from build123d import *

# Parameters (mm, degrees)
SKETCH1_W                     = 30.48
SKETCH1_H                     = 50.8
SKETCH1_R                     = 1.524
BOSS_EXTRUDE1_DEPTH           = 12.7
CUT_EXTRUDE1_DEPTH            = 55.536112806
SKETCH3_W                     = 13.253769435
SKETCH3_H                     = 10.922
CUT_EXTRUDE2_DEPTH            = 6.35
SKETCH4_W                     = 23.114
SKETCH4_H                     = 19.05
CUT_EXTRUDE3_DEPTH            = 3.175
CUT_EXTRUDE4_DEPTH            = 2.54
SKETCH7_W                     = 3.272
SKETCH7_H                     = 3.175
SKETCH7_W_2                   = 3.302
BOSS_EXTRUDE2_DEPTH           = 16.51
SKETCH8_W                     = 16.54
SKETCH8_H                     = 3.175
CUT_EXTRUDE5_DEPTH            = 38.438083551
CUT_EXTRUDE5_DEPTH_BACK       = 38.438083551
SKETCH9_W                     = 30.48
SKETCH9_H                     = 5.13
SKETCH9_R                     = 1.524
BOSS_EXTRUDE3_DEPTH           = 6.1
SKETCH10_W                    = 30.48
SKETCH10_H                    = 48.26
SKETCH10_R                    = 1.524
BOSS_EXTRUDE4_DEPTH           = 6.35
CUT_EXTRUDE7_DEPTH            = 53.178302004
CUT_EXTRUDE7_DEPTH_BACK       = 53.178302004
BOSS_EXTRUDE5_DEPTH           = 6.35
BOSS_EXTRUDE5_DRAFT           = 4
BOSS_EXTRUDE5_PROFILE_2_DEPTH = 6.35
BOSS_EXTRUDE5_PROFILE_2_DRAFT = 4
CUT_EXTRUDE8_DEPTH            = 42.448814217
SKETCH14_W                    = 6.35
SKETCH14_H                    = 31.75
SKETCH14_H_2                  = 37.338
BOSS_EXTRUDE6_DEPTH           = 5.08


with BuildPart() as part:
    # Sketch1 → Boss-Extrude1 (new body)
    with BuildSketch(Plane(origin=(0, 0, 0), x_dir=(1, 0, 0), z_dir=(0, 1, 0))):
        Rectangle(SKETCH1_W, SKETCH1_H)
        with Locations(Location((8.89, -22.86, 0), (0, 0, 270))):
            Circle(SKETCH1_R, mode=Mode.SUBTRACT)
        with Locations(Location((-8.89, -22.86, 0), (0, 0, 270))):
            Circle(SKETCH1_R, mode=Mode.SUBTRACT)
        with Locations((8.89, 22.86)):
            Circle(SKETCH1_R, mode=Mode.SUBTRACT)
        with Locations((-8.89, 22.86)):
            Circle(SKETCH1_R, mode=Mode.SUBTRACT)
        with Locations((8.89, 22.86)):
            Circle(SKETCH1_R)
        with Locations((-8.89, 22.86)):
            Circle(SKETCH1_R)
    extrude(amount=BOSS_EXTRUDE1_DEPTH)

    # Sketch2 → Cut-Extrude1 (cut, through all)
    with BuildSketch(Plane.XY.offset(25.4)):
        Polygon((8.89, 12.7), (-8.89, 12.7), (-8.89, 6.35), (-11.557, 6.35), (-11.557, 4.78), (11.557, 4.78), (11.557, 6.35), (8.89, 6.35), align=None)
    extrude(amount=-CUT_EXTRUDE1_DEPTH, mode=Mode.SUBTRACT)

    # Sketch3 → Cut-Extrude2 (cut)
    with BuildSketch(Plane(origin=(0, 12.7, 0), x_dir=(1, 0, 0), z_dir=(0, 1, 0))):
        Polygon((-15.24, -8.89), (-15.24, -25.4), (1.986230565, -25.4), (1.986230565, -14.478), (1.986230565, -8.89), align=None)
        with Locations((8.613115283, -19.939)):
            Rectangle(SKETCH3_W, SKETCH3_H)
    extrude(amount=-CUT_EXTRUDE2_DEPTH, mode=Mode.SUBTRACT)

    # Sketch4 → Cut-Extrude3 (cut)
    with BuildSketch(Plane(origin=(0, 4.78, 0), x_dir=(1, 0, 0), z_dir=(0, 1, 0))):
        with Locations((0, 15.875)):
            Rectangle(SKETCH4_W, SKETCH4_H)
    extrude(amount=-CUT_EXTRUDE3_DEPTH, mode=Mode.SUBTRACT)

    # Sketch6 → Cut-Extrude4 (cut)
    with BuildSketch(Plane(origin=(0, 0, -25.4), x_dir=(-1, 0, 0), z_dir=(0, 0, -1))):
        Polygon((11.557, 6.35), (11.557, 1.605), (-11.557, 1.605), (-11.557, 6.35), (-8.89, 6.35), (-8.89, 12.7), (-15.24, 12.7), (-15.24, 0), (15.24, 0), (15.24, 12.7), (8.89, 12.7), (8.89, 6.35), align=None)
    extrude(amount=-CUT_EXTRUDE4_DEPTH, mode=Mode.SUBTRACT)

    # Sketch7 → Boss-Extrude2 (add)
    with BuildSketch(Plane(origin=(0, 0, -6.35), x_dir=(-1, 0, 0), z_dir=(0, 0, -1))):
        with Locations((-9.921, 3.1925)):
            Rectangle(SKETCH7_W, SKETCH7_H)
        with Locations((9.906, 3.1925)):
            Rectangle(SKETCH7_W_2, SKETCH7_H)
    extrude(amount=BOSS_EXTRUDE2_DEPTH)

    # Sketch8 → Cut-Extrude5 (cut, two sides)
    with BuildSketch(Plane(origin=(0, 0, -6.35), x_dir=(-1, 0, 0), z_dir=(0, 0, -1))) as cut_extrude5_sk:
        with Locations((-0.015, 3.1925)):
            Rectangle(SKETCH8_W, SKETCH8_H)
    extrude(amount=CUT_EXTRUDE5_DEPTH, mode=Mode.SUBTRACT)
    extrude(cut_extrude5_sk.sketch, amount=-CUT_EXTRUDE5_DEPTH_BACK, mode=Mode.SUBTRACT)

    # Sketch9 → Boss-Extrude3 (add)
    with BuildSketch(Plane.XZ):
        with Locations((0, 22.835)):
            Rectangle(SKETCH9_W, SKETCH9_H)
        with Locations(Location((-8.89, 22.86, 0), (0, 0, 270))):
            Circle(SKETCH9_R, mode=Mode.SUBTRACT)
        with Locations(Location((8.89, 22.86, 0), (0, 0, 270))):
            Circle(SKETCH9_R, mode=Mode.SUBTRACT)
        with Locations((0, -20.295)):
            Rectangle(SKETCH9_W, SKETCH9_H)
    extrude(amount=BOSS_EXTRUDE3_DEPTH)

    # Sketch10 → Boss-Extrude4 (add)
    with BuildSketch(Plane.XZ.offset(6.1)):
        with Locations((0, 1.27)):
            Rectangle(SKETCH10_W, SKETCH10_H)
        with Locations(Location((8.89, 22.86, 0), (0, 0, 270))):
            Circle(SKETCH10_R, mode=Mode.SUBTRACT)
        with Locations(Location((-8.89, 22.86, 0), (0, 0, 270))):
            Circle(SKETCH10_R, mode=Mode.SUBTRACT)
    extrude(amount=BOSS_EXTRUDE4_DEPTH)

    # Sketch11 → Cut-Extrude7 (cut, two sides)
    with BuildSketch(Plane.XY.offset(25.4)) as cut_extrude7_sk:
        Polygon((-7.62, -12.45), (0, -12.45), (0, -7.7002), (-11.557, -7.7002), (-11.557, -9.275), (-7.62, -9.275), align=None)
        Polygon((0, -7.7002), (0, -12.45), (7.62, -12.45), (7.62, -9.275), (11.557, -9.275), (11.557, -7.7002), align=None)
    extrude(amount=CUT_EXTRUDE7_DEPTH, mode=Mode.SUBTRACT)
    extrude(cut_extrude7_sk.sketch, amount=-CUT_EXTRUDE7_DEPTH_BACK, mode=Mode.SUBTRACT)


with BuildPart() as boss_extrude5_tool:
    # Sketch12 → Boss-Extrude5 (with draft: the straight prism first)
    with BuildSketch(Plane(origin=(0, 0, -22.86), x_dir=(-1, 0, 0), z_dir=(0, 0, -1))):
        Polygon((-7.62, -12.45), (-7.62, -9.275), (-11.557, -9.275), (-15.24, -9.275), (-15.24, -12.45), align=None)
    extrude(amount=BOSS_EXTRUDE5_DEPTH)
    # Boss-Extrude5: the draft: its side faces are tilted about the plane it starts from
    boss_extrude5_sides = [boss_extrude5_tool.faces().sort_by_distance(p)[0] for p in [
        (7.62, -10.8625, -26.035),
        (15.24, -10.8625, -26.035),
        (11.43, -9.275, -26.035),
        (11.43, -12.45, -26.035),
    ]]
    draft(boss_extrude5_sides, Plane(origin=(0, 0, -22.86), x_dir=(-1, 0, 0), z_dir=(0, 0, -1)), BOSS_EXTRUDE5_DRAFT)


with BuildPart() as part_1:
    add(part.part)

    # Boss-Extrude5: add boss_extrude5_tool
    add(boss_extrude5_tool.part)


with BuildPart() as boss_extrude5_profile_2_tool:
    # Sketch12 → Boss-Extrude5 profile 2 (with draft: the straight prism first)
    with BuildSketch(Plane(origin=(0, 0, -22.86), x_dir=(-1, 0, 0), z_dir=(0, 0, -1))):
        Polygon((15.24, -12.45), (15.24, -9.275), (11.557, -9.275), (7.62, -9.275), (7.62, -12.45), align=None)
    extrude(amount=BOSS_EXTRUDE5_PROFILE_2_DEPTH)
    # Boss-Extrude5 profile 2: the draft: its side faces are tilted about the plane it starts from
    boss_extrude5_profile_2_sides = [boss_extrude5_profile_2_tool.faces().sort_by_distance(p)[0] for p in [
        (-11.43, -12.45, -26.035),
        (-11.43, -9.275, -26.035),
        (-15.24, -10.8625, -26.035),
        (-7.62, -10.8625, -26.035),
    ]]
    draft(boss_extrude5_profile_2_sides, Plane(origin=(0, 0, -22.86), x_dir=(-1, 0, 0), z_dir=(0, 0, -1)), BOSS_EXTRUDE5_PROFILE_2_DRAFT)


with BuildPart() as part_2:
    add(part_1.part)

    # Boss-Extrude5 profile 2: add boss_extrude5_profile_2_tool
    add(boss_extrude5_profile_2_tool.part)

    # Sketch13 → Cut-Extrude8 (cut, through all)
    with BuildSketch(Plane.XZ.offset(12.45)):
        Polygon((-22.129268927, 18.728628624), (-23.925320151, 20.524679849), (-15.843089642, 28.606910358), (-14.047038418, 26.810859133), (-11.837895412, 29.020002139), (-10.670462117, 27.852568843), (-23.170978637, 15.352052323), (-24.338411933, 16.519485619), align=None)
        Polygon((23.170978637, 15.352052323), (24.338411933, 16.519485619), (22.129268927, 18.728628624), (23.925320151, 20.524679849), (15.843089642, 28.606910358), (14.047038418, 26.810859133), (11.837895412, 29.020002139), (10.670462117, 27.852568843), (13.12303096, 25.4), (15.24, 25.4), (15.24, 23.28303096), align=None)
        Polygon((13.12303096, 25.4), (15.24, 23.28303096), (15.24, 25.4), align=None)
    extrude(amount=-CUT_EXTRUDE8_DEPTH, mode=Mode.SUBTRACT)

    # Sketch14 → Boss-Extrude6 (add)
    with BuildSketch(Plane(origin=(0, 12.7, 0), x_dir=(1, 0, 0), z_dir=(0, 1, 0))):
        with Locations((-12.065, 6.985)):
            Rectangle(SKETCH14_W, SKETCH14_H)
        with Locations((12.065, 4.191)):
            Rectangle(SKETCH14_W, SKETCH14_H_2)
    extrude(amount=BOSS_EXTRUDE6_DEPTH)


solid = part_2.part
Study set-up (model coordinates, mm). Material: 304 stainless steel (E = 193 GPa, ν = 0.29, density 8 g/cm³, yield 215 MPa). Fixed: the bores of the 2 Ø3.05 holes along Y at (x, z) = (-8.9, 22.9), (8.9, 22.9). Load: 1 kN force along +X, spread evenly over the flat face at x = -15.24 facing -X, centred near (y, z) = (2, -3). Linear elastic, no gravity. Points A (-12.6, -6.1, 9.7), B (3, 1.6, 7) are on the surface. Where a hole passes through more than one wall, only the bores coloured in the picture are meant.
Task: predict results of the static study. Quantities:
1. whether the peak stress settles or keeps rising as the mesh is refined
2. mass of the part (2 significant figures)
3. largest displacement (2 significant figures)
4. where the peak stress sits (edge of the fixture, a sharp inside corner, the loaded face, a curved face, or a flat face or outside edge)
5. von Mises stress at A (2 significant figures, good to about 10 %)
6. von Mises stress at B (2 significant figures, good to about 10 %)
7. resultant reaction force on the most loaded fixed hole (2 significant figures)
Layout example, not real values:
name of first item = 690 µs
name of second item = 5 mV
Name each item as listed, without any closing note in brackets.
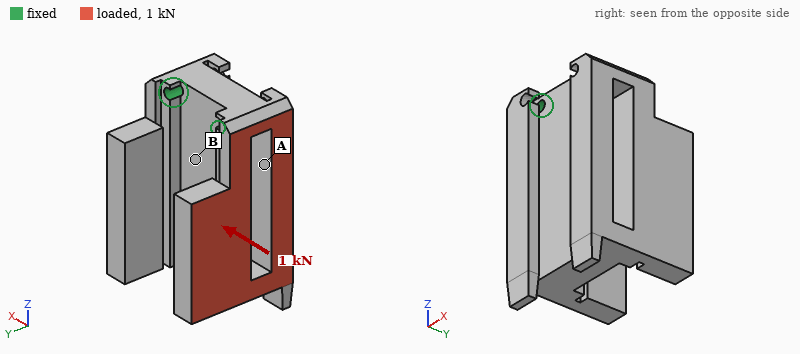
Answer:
whether the peak stress settles or keeps rising as the mesh is refined = keeps rising
mass of the part = 140 g
largest displacement = 46 µm
where the peak stress sits = edge of the fixture
von Mises stress at A = 9.1 MPa
von Mises stress at B = 28 MPa
resultant reaction force on the most loaded fixed hole = 1.2 kN
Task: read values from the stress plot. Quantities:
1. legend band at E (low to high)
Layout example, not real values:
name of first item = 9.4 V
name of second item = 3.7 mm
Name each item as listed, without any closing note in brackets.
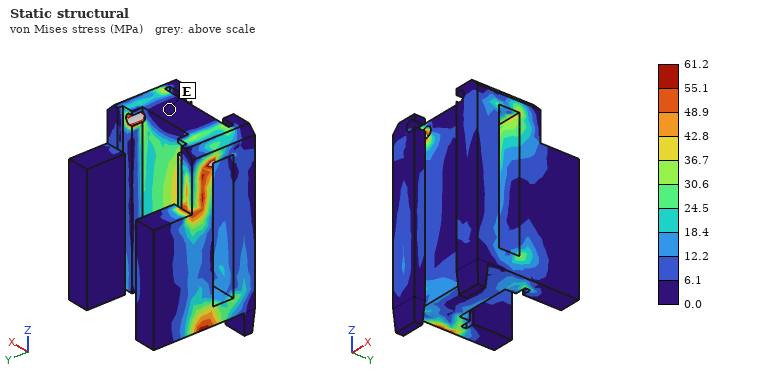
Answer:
legend band at E = 0.0 to 6.1 MPa
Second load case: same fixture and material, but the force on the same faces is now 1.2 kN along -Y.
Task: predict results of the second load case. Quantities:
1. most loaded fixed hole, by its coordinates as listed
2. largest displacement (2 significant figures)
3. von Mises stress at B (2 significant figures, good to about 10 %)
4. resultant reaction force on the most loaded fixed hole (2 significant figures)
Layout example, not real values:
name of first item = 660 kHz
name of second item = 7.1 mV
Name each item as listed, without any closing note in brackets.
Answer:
most loaded fixed hole, by its coordinates as listed = (-8.9, 22.9)
largest displacement = 0.14 mm
von Mises stress at B = 45 MPa
resultant reaction force on the most loaded fixed hole = 1.1 kN
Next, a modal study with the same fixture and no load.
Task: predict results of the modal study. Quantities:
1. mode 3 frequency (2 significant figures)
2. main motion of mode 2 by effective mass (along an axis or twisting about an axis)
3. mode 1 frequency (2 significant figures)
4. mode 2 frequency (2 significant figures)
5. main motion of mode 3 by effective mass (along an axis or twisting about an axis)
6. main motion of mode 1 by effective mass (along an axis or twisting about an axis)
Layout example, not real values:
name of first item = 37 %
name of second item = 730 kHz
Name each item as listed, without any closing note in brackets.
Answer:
mode 3 frequency = 5000 Hz
main motion of mode 2 by effective mass = along X
mode 1 frequency = 1900 Hz
mode 2 frequency = 2800 Hz
main motion of mode 3 by effective mass = along X
main motion of mode 1 by effective mass = along Y
